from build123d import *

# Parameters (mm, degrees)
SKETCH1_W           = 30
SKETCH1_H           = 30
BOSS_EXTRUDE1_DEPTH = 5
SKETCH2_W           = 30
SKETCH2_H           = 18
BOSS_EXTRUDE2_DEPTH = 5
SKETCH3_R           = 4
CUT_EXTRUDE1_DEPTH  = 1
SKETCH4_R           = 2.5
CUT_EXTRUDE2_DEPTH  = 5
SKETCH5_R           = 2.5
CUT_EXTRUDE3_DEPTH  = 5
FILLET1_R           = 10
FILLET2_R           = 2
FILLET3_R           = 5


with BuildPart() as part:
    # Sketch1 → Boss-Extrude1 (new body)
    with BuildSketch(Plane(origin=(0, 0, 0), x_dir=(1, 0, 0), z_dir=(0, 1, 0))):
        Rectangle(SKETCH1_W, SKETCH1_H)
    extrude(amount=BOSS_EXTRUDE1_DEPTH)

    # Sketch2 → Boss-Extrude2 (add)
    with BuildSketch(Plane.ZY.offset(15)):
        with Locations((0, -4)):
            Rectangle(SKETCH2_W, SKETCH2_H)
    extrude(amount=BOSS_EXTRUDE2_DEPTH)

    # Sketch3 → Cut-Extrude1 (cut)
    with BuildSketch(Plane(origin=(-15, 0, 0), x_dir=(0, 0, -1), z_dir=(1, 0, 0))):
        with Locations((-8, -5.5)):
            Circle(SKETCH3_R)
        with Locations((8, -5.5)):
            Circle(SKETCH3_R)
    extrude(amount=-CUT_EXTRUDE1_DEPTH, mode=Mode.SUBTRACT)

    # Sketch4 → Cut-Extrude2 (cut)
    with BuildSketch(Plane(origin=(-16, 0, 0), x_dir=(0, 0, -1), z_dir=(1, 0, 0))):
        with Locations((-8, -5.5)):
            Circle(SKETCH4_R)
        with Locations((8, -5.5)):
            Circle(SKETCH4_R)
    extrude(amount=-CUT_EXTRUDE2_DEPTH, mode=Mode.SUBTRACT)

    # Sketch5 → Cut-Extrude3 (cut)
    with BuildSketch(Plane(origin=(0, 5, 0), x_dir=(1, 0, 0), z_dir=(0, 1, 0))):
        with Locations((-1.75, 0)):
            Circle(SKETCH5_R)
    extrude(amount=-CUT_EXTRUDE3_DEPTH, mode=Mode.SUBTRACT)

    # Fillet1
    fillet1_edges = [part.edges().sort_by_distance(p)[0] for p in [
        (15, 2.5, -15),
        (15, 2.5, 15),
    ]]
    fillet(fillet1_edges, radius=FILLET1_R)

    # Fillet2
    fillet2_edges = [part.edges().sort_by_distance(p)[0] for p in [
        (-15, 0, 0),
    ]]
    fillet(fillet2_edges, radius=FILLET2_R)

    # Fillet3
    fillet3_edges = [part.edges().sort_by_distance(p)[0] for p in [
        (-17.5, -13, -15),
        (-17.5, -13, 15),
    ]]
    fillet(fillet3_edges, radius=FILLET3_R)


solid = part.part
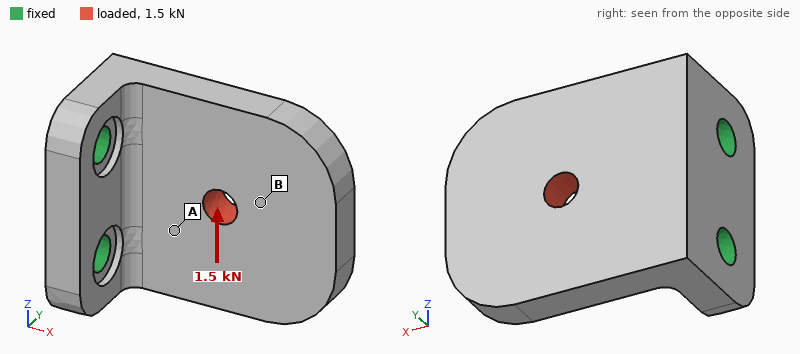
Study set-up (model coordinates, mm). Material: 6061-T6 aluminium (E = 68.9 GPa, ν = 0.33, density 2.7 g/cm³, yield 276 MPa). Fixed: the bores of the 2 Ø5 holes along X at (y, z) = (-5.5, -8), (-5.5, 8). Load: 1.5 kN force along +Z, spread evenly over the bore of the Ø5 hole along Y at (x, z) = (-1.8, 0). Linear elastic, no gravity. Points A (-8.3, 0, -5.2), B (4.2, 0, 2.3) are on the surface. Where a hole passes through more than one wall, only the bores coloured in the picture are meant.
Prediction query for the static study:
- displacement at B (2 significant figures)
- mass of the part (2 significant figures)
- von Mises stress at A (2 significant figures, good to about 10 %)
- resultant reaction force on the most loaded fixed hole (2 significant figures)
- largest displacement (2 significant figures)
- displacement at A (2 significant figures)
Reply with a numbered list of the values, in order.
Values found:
1. 46 µm
2. 18 g
3. 37 MPa
4. 1.6 kN
5. 64 µm
6. 23 µm
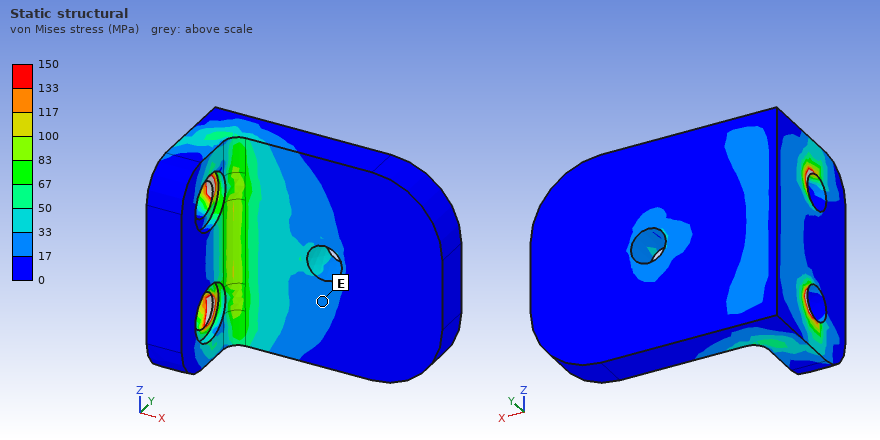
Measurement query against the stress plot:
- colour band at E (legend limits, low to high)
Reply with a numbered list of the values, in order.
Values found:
1. 17 to 33 MPa
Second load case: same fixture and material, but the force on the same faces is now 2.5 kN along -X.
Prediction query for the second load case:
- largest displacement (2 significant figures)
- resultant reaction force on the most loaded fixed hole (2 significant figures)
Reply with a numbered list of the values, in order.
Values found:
1. 0.14 mm
2. 1.3 kN
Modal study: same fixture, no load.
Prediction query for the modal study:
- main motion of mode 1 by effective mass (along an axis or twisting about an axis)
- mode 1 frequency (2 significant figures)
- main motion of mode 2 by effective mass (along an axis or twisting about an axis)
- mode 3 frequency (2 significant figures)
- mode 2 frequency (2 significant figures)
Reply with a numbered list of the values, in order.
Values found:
1. along Y
2. 3200 Hz
3. along Z
4. 11 kHz
5. 7500 Hz
